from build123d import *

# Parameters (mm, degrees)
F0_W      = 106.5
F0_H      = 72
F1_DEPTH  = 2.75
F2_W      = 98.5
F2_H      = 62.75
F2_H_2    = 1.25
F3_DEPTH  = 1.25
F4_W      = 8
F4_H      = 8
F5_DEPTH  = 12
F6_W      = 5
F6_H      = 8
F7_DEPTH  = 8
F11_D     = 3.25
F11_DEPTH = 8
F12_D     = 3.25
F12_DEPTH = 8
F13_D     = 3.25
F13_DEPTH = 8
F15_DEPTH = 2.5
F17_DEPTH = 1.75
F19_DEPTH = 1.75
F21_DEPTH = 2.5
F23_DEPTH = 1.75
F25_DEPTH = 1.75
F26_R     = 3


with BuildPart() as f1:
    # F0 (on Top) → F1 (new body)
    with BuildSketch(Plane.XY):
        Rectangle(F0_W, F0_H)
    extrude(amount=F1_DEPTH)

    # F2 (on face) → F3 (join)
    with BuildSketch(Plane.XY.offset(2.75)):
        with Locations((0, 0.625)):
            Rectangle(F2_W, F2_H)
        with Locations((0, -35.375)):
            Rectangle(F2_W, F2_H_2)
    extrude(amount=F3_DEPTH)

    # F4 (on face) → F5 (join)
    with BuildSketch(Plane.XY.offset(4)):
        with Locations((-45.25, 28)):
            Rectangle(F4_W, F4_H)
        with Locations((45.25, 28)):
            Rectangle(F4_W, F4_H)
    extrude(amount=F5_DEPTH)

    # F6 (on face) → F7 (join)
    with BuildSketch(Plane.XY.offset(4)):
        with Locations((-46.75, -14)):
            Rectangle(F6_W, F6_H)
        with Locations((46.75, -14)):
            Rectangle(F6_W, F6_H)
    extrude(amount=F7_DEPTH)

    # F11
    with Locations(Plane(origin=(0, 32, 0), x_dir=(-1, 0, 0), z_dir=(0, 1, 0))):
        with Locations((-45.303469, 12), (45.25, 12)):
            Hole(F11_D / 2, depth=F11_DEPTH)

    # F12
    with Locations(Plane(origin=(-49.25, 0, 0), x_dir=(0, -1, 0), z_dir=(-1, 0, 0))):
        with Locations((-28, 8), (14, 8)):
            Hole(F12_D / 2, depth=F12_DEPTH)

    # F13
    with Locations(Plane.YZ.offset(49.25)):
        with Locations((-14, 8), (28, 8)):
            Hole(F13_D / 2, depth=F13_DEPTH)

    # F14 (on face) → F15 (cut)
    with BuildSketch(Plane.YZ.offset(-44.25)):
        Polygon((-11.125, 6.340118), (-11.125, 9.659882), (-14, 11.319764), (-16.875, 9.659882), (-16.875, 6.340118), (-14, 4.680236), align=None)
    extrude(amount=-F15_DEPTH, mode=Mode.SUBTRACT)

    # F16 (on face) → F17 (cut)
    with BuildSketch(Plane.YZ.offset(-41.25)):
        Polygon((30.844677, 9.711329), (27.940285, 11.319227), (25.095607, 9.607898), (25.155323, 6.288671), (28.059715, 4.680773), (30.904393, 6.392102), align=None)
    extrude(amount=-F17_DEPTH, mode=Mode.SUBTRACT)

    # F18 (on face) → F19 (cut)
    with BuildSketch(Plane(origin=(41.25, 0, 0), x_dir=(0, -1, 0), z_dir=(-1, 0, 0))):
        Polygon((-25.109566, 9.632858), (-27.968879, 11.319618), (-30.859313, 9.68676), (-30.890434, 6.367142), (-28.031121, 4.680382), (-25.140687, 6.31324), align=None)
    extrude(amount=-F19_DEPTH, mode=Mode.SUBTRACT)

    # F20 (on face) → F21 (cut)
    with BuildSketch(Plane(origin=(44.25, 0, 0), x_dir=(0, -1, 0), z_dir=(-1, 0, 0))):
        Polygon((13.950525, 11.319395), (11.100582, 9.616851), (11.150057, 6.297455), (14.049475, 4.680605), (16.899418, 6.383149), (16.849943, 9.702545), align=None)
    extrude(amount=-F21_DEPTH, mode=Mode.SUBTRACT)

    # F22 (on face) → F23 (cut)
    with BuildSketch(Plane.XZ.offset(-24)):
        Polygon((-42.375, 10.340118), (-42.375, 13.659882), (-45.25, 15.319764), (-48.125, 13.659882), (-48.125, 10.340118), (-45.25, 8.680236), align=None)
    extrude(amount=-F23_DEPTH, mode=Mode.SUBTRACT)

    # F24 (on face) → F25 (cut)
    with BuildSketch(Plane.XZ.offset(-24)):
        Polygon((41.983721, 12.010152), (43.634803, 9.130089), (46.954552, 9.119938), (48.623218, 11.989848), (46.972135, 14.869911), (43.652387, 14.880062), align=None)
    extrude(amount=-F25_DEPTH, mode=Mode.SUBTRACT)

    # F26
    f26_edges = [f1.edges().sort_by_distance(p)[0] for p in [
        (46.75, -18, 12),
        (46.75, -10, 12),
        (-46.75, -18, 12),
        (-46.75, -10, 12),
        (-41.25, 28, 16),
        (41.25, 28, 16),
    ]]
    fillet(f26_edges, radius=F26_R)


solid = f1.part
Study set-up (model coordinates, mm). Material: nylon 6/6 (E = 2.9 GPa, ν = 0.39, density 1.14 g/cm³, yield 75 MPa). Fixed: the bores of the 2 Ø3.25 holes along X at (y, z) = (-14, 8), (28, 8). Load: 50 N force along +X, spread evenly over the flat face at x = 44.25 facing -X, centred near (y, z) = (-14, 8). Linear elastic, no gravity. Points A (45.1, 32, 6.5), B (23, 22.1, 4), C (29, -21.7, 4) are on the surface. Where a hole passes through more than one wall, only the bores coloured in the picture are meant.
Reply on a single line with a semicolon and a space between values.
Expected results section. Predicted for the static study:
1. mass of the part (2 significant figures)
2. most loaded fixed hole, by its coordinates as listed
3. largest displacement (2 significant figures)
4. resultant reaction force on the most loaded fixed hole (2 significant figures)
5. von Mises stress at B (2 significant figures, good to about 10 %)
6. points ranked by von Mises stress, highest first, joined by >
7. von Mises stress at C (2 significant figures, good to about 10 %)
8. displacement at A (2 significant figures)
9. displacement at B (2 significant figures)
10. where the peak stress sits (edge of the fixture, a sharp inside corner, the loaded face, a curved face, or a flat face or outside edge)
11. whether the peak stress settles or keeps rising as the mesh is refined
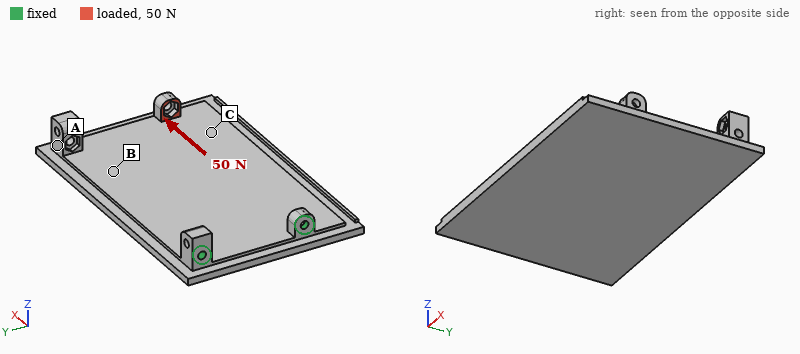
35 g; (-14, 8); 1.4 mm; 49 N; 1.3 MPa; C > B > A; 2.4 MPa; 1.0 mm; 0.65 mm; edge of the fixture; keeps rising
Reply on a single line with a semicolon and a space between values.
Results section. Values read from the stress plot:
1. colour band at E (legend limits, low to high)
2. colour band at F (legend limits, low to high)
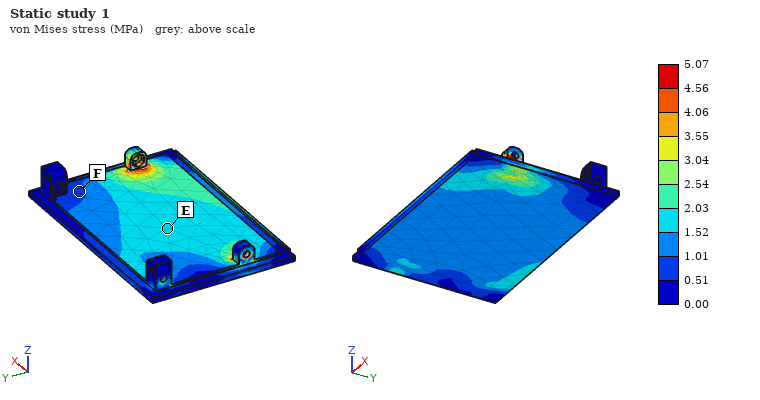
1.52 to 2.03 MPa; 0.51 to 1.01 MPa
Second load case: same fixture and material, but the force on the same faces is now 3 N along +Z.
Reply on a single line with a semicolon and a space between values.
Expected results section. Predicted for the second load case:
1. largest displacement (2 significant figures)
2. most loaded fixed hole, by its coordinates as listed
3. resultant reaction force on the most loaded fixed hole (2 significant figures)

1.3 mm; (-14, 8); 3.6 N
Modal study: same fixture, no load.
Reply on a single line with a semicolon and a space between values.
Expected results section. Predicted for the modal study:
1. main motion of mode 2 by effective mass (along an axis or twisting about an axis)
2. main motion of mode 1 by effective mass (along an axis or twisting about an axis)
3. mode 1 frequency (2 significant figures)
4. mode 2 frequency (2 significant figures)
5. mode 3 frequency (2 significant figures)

twisting about X; along Z; 80 Hz; 280 Hz; 530 Hz
